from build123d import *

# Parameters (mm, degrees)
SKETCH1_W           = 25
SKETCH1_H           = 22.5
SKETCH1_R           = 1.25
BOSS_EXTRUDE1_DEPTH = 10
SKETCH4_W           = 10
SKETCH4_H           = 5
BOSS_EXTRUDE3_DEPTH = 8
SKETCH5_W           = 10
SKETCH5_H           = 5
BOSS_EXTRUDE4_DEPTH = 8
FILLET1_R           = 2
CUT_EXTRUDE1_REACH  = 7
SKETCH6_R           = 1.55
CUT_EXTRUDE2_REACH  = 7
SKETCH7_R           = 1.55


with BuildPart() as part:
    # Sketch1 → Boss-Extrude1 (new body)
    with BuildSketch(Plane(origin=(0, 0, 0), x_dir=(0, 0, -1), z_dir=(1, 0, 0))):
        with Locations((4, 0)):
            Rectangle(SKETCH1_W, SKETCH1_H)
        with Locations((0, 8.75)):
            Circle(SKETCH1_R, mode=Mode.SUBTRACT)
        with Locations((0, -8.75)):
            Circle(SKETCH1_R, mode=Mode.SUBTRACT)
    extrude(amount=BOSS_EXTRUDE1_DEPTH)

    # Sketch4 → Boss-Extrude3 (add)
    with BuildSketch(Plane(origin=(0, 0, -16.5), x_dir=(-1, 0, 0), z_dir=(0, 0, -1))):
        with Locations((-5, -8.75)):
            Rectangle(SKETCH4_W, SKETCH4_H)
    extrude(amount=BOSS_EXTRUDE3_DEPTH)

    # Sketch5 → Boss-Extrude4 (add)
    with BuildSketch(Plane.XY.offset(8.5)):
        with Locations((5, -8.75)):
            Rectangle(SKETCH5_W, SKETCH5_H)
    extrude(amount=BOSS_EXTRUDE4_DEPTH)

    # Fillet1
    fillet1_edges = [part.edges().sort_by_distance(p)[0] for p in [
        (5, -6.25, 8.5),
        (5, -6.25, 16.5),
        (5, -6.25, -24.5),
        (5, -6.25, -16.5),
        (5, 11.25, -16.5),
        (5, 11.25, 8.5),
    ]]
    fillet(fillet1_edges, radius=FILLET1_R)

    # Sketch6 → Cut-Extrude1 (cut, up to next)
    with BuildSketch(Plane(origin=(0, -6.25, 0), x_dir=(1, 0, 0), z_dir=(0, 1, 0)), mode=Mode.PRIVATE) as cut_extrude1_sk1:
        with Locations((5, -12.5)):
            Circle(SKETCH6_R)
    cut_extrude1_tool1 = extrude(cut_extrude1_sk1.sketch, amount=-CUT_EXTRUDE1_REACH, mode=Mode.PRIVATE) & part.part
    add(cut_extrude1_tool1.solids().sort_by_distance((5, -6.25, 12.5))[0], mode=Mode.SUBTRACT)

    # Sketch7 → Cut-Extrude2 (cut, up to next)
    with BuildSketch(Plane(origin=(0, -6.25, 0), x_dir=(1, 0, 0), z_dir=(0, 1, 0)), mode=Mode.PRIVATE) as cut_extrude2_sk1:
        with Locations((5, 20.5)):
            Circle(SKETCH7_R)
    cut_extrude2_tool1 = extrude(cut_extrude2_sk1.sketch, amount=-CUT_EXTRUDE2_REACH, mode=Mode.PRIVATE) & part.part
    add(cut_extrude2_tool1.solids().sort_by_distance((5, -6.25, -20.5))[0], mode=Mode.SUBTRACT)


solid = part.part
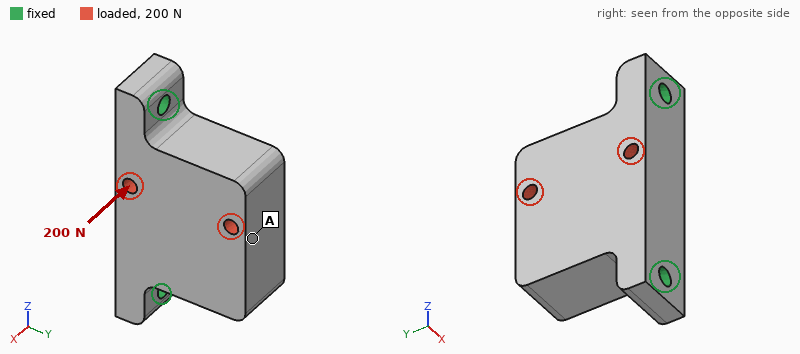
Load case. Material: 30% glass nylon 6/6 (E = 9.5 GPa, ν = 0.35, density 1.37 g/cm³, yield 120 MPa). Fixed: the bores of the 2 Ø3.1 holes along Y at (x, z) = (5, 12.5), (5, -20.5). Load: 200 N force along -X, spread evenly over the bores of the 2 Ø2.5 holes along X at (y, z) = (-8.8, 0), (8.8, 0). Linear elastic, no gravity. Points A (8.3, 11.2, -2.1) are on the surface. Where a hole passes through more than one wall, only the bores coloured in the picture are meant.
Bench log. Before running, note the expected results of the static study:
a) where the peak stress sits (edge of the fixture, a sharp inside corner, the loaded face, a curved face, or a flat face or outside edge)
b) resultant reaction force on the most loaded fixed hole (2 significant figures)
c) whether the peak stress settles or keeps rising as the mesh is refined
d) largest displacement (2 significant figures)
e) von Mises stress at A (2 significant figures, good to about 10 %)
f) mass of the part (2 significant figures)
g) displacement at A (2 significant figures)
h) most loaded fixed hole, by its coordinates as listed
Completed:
edge of the fixture
130 N
keeps rising
98 µm
2.4 MPa
8.5 g
95 µm
(5, 12.5)
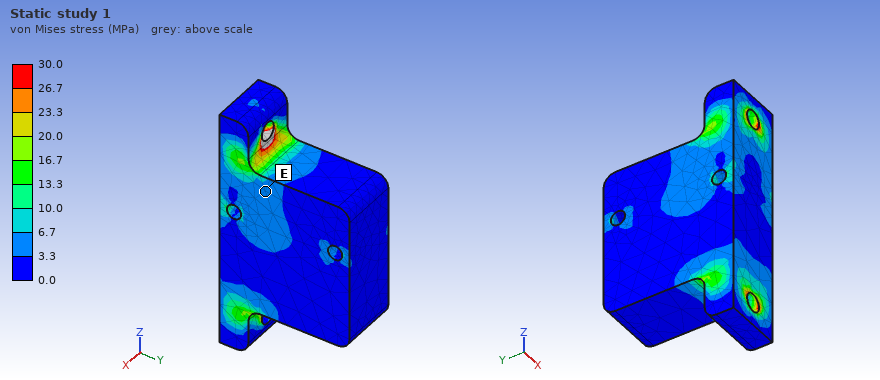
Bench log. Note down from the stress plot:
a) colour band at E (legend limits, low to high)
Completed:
3.3 to 6.7 MPa
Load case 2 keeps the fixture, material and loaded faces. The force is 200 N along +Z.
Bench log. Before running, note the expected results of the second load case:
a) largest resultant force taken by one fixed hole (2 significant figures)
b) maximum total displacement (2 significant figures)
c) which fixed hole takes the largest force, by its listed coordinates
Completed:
120 N
8.2 µm
(5, 12.5)
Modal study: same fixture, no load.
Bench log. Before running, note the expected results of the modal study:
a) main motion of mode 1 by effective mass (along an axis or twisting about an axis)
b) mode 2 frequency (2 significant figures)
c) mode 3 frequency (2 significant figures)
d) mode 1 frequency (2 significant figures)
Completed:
along X
11 kHz
11 kHz
3300 Hz
